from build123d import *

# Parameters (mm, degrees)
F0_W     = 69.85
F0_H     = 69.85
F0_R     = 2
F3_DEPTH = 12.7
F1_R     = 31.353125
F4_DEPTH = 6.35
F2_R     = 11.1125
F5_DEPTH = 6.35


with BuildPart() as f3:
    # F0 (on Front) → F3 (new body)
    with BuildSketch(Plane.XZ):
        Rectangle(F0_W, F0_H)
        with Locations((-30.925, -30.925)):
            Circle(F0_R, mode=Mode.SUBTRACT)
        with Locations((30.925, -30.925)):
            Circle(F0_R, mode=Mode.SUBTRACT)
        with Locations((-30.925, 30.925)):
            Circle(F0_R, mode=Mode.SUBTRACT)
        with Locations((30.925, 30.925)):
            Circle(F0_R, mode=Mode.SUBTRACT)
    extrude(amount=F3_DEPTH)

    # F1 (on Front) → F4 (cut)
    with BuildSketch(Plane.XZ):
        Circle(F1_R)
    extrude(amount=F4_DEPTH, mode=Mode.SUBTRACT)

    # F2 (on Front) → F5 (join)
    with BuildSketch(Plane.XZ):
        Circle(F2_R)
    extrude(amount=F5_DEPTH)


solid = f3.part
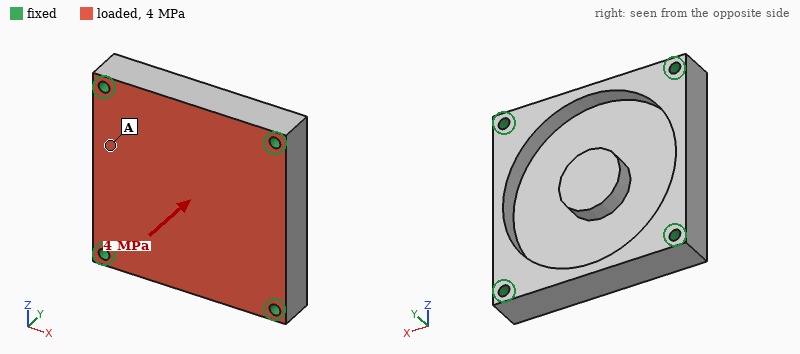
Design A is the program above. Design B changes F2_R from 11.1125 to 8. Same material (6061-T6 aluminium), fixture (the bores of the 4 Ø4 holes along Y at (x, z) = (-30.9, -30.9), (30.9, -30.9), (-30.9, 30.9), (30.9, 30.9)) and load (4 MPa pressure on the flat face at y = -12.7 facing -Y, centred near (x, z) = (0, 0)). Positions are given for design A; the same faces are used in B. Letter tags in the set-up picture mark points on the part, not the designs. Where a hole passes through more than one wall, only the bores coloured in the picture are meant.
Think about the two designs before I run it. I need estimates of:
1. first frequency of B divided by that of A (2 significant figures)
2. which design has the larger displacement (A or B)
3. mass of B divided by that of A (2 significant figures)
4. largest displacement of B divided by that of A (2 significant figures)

1.0
B
0.97
1.1
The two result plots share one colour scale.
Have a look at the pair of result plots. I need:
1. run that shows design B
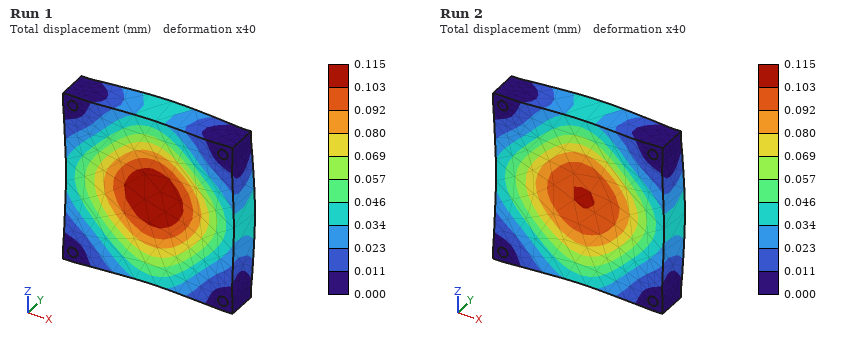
Run 1
